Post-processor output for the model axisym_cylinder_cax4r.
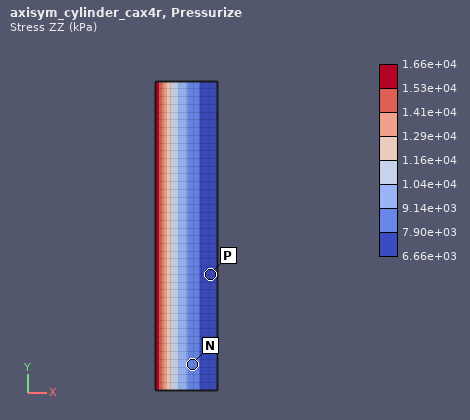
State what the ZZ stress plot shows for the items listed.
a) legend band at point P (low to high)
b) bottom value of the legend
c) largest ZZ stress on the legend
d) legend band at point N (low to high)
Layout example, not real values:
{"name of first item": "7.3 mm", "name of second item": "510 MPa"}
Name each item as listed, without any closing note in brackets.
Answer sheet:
{"legend band at point P": "6.66e+03 to 7.90e+03 kPa", "bottom value of the legend": "6.66e+03 kPa", "largest ZZ stress on the legend": "1.66e+04 kPa", "legend band at point N": "7.90e+03 to 9.14e+03 kPa"}
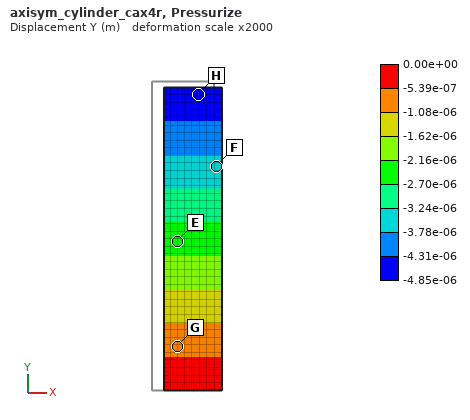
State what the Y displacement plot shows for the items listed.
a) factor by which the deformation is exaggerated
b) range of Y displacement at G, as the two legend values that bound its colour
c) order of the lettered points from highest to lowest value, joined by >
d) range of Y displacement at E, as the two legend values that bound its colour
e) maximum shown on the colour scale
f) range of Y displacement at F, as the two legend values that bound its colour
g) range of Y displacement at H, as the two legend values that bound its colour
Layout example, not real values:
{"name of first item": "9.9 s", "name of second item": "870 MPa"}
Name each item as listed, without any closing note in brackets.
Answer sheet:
{"factor by which the deformation is exaggerated": "2000", "range of Y displacement at G, as the two legend values that bound its colour": "-1.08e-06 to -5.39e-07 m", "order of the lettered points from highest to lowest value, joined by >": "G > E > F > H", "range of Y displacement at E, as the two legend values that bound its colour": "-2.70e-06 to -2.16e-06 m", "maximum shown on the colour scale": "0.00e+00 m", "range of Y displacement at F, as the two legend values that bound its colour": "-3.78e-06 to -3.24e-06 m", "range of Y displacement at H, as the two legend values that bound its colour": "-4.85e-06 to -4.31e-06 m"}
